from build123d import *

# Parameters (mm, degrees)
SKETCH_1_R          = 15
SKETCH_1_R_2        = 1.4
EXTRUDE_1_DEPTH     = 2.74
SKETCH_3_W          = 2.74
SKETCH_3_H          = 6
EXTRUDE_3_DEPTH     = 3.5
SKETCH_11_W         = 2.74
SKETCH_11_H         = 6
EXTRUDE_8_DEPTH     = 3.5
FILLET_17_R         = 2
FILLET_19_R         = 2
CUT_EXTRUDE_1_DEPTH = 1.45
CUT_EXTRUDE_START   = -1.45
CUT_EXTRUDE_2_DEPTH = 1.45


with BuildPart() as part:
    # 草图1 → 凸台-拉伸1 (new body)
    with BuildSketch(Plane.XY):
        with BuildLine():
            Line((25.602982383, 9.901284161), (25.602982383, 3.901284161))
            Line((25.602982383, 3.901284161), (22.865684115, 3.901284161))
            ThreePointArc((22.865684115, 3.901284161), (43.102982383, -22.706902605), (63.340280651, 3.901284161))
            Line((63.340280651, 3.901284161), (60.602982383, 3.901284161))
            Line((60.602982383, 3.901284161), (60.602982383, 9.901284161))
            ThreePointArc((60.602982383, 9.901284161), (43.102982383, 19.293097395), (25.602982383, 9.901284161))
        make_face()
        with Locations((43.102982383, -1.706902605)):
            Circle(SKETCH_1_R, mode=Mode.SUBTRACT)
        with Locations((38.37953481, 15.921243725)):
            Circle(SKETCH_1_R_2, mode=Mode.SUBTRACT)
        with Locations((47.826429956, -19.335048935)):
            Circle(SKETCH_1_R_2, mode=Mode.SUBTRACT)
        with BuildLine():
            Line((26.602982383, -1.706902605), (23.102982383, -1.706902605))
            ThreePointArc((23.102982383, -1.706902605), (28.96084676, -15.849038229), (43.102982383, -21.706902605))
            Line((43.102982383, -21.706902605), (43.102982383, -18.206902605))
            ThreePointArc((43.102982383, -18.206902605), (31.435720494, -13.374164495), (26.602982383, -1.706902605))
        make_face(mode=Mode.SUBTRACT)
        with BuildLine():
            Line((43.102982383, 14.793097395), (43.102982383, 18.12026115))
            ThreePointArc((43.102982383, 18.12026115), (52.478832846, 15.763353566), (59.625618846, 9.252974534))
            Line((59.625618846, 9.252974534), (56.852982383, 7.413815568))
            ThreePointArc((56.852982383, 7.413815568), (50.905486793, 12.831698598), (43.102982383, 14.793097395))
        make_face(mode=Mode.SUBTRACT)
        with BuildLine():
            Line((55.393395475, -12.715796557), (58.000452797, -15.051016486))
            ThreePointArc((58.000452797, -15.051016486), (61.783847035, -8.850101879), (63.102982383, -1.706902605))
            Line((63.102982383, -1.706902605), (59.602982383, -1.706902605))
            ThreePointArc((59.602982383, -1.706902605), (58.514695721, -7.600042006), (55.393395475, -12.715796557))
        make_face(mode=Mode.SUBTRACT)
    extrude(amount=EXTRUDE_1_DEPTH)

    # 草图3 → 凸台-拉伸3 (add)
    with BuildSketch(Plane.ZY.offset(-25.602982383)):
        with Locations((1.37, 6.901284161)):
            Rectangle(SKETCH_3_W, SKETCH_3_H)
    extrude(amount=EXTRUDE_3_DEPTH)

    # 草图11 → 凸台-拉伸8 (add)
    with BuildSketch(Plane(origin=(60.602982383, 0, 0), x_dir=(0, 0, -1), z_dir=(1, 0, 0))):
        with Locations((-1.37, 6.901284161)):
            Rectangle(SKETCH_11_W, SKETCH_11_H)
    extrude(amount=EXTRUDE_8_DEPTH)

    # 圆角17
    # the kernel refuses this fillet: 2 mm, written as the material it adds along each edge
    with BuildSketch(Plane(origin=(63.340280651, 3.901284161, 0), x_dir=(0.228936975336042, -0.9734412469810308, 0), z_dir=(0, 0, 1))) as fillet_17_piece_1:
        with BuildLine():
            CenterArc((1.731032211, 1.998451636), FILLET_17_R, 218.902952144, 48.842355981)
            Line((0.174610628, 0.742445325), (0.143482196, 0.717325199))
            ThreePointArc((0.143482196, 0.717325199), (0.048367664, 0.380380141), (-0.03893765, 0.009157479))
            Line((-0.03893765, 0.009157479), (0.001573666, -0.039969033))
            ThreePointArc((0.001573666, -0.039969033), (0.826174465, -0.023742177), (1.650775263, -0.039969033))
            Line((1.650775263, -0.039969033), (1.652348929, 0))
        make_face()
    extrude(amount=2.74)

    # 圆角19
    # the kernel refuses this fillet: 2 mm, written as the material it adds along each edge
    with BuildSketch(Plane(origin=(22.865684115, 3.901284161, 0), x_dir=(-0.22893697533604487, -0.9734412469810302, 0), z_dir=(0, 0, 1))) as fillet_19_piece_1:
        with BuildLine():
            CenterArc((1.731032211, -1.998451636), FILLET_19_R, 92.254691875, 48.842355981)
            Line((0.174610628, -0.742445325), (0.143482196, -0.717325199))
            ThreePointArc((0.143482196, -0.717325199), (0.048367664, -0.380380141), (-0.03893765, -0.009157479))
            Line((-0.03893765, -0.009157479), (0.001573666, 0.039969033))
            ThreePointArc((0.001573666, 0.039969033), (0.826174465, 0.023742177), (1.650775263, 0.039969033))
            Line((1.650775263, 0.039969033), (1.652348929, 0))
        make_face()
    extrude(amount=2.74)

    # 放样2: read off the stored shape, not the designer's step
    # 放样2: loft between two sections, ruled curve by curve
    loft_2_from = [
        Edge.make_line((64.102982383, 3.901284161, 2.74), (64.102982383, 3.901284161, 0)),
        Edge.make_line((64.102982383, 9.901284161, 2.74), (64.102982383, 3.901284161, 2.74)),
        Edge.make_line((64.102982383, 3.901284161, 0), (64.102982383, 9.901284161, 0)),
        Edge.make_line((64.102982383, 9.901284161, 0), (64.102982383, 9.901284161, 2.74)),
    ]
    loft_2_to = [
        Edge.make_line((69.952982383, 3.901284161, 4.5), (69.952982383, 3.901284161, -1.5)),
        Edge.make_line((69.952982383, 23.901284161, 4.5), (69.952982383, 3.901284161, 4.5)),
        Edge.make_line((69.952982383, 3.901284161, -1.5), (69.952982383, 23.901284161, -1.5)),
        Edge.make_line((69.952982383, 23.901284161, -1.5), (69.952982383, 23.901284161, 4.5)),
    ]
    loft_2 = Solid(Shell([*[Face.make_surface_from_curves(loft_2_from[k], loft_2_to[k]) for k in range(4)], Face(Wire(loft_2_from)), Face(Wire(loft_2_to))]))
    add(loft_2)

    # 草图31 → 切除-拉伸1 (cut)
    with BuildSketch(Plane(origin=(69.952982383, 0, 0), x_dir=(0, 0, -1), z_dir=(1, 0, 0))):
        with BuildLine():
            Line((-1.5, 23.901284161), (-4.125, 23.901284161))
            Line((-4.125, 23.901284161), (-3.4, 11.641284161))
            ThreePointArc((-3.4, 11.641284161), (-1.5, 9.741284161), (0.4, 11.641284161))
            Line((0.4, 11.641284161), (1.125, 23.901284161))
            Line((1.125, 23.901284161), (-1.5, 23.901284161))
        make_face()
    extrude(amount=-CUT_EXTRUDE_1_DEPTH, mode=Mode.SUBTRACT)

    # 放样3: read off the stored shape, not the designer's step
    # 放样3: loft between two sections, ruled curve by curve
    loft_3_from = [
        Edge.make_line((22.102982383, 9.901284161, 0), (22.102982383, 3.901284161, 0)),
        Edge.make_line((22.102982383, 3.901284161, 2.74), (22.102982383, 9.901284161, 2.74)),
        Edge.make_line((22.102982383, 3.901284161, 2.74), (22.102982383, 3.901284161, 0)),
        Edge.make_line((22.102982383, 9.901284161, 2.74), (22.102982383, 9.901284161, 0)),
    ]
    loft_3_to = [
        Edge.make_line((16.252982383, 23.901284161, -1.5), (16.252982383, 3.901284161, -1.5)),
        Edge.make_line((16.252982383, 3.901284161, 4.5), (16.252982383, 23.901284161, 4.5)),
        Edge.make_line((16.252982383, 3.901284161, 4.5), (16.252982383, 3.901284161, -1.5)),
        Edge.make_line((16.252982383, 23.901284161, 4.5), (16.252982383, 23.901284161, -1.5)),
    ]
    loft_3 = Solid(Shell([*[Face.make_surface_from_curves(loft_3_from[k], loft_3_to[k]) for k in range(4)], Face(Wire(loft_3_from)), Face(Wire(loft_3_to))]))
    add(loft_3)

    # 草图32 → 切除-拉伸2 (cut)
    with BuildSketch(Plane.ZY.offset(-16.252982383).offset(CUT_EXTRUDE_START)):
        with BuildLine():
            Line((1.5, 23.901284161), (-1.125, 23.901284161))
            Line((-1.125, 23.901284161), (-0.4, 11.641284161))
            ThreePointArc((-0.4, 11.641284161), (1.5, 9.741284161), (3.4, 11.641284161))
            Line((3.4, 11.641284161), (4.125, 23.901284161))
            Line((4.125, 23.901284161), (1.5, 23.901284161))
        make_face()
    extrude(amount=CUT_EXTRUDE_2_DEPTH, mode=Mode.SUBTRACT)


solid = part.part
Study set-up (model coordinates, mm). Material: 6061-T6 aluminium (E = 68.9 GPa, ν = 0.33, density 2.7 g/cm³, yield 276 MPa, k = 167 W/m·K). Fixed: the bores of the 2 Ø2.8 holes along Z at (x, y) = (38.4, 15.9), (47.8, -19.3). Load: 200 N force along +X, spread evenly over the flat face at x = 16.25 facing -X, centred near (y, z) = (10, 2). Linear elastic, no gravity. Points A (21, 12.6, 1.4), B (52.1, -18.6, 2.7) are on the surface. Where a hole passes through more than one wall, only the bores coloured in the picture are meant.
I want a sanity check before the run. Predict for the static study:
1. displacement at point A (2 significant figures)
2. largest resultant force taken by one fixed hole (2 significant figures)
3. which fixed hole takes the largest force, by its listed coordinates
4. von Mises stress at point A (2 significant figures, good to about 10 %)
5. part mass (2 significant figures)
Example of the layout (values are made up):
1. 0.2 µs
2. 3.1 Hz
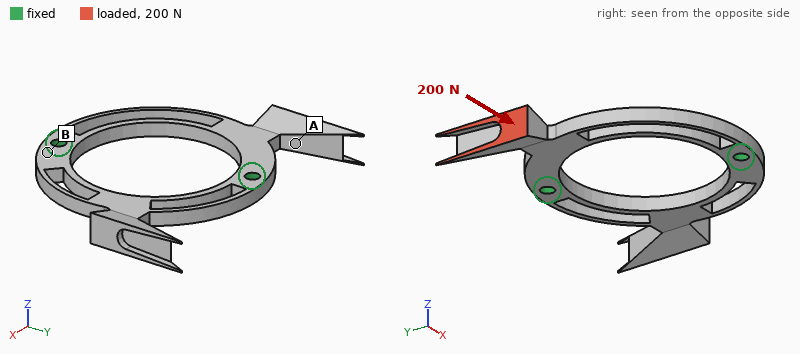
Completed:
1. 21 µm
2. 190 N
3. (38.4, 15.9)
4. 23 MPa
5. 5.1 g
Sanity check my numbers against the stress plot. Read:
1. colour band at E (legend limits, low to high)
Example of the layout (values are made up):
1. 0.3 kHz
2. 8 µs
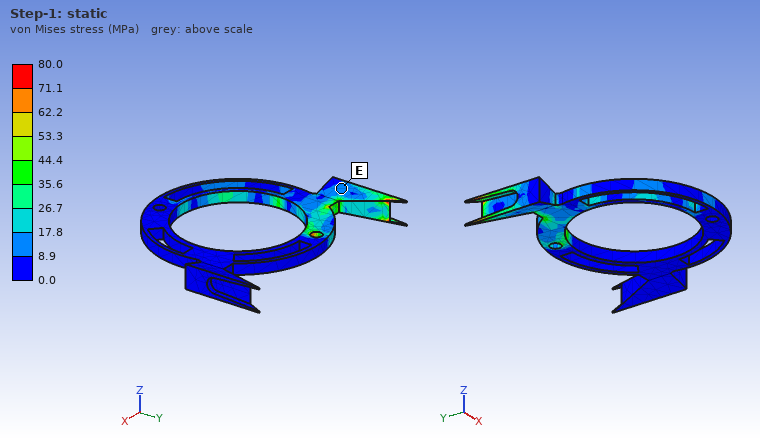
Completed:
1. 8.9 to 17.8 MPa
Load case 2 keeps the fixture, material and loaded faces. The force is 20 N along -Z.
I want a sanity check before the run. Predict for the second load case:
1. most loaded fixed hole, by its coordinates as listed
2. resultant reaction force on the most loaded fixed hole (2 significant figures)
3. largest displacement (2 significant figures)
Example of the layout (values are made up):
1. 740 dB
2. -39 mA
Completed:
1. (38.4, 15.9)
2. 19 N
3. 0.12 mm
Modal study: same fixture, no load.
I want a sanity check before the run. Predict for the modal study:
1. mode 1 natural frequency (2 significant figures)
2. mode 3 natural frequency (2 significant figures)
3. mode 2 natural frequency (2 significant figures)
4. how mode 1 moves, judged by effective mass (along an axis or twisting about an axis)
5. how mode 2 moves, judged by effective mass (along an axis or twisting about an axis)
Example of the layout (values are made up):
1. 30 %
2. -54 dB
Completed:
1. 1500 Hz
2. 5500 Hz
3. 2600 Hz
4. along Z
5. along Z
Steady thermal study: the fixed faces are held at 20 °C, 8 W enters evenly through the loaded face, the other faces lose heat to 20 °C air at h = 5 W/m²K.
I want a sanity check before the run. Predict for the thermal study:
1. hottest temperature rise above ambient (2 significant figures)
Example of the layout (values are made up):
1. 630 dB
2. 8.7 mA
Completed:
1. 71 K
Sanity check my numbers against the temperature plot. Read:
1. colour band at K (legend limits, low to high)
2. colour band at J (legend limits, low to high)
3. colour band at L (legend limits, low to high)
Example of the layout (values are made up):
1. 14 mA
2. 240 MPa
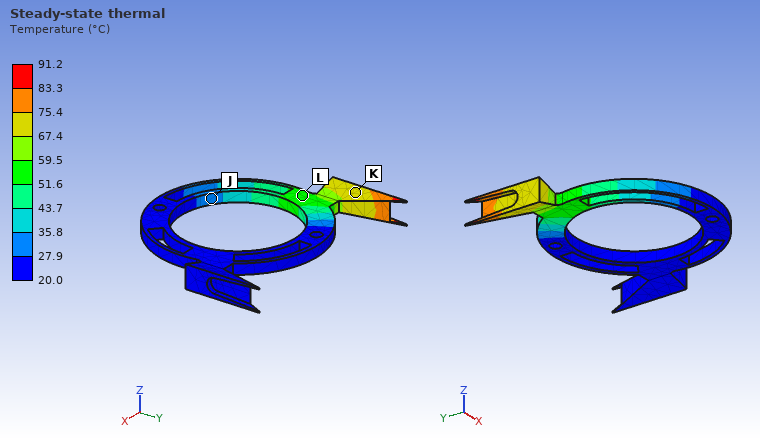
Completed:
1. 67.4 to 75.4 °C
2. 27.9 to 35.8 °C
3. 51.6 to 59.5 °C
